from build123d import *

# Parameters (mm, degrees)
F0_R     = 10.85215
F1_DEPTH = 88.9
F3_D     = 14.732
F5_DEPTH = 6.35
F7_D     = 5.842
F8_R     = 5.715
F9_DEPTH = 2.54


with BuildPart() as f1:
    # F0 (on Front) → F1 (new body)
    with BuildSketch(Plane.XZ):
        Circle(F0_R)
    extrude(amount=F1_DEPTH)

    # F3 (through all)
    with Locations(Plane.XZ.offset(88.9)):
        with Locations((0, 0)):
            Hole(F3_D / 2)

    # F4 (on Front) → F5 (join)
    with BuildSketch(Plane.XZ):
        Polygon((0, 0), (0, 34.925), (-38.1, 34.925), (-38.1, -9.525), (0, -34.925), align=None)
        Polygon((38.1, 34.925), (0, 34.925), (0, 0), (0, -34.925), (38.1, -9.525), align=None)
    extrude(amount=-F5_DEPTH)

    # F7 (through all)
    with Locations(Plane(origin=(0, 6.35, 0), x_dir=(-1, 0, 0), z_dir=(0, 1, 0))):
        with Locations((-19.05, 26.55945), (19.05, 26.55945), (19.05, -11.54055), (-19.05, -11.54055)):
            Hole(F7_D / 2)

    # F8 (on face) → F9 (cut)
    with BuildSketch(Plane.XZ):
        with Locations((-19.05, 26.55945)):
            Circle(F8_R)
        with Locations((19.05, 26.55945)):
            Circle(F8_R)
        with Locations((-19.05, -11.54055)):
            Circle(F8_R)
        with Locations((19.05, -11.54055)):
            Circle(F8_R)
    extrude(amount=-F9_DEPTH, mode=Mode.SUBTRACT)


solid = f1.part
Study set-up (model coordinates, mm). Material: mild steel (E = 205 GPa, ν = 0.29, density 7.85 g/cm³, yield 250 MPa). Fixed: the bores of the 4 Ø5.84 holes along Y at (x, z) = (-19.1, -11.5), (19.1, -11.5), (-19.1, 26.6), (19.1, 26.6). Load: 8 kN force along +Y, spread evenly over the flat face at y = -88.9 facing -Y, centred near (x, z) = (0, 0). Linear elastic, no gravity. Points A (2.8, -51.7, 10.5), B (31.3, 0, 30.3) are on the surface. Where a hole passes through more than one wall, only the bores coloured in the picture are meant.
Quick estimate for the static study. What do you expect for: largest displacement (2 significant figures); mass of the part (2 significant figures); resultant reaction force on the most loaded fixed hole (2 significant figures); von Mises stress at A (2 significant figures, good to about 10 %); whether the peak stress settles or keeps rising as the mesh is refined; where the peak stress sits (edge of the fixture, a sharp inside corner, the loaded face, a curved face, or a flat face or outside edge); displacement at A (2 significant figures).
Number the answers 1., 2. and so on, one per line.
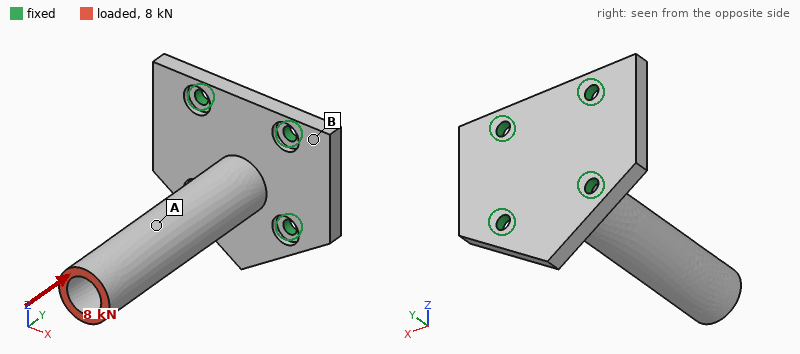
1. 47 µm
2. 340 g
3. 3.4 kN
4. 40 MPa
5. keeps rising
6. edge of the fixture
7. 35 µm
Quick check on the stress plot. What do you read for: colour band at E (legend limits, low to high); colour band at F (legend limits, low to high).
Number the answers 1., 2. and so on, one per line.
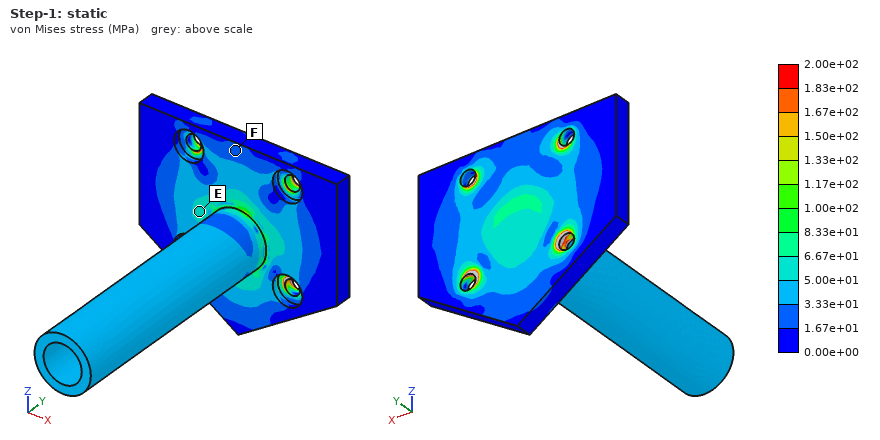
1. 5.00e+01 to 6.67e+01 MPa
2. 1.67e+01 to 3.33e+01 MPa
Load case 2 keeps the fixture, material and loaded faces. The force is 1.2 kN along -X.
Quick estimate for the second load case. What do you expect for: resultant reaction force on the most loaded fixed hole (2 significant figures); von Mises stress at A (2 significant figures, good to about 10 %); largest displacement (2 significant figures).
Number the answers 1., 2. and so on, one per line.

1. 2.7 kN
2. 23 MPa
3. 0.27 mm
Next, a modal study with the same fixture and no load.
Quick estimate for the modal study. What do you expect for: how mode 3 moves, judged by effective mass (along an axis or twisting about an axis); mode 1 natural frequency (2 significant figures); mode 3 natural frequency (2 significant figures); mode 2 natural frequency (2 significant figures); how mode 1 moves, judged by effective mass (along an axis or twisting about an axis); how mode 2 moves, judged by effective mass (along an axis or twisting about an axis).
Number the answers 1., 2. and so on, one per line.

1. along Y
2. 1600 Hz
3. 7200 Hz
4. 1700 Hz
5. along Z
6. along X
